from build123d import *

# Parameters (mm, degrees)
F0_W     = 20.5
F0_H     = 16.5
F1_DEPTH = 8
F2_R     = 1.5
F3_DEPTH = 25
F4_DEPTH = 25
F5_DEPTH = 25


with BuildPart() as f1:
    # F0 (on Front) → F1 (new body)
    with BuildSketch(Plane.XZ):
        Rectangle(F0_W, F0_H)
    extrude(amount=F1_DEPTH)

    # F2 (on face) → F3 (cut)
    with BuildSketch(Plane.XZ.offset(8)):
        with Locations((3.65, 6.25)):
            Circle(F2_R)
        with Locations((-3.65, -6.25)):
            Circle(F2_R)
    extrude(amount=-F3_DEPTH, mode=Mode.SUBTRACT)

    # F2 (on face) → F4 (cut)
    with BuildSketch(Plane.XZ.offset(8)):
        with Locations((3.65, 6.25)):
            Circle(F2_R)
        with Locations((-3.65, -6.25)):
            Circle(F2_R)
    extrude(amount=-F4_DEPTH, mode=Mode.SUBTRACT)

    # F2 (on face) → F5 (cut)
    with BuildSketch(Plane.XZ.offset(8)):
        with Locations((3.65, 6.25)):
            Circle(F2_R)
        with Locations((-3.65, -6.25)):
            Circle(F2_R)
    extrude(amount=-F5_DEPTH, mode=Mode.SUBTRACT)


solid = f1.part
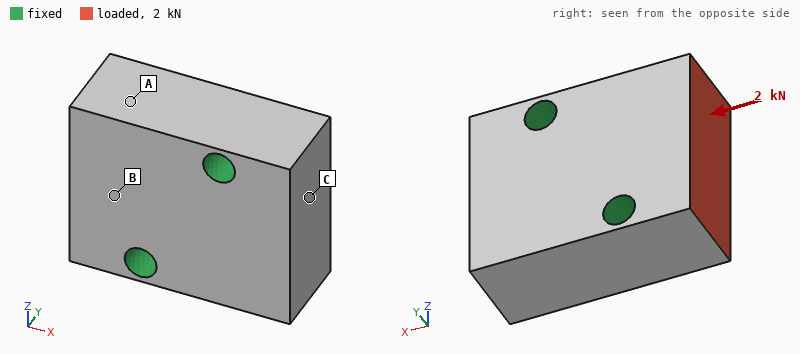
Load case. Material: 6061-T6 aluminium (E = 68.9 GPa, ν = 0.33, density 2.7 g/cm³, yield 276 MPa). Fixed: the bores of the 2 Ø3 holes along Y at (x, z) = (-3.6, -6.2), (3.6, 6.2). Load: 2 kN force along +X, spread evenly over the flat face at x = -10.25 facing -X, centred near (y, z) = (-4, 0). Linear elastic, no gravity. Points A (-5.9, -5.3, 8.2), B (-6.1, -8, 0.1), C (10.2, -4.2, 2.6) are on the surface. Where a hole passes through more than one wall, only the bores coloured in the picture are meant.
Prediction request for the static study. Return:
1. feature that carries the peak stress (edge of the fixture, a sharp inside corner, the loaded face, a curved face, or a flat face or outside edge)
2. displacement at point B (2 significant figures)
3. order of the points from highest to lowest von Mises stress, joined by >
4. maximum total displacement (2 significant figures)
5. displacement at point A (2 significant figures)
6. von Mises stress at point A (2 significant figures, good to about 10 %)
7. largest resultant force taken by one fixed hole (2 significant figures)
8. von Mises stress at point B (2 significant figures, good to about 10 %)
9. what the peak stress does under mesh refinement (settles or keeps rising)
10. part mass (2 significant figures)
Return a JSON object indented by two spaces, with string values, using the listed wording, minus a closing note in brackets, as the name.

{
  "feature that carries the peak stress": "edge of the fixture",
  "displacement at point B": "1.9 µm",
  "order of the points from highest to lowest von Mises stress, joined by >": "A > B > C",
  "maximum total displacement": "3.9 µm",
  "displacement at point A": "2.8 µm",
  "von Mises stress at point A": "17 MPa",
  "largest resultant force taken by one fixed hole": "1.0 kN",
  "von Mises stress at point B": "12 MPa",
  "what the peak stress does under mesh refinement": "keeps rising",
  "part mass": "7.0 g"
}
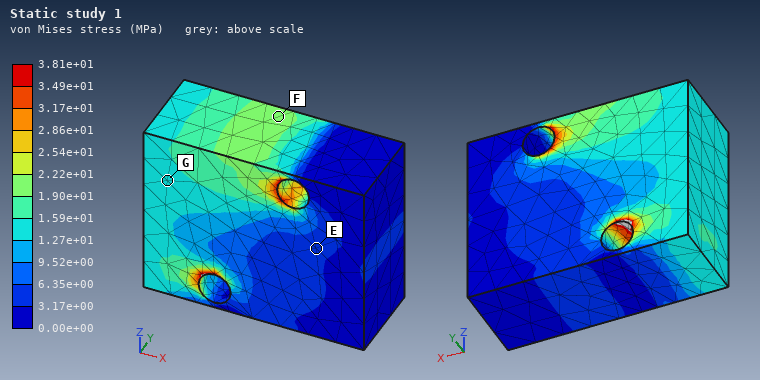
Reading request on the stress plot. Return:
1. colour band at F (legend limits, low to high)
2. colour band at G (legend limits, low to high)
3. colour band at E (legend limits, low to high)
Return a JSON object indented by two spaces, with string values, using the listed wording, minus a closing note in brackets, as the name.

{
  "colour band at F": "1.90e+01 to 2.22e+01 MPa",
  "colour band at G": "1.27e+01 to 1.59e+01 MPa",
  "colour band at E": "3.17e+00 to 6.35e+00 MPa"
}
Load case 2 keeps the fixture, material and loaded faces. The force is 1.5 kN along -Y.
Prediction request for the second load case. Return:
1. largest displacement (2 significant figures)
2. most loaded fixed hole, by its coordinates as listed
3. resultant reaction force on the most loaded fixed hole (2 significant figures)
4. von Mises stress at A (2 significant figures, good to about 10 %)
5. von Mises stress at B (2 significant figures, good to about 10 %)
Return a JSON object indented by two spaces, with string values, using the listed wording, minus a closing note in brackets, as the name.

{
  "largest displacement": "22 µm",
  "most loaded fixed hole, by its coordinates as listed": "(-3.6, -6.2)",
  "resultant reaction force on the most loaded fixed hole": "1.2 kN",
  "von Mises stress at A": "28 MPa",
  "von Mises stress at B": "32 MPa"
}
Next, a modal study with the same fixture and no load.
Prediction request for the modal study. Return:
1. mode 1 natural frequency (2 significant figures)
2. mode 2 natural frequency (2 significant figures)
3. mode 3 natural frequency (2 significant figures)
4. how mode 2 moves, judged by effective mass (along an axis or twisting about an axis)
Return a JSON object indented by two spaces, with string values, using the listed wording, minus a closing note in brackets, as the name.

{
  "mode 1 natural frequency": "38 kHz",
  "mode 2 natural frequency": "46 kHz",
  "mode 3 natural frequency": "71 kHz",
  "how mode 2 moves, judged by effective mass": "along Y"
}
